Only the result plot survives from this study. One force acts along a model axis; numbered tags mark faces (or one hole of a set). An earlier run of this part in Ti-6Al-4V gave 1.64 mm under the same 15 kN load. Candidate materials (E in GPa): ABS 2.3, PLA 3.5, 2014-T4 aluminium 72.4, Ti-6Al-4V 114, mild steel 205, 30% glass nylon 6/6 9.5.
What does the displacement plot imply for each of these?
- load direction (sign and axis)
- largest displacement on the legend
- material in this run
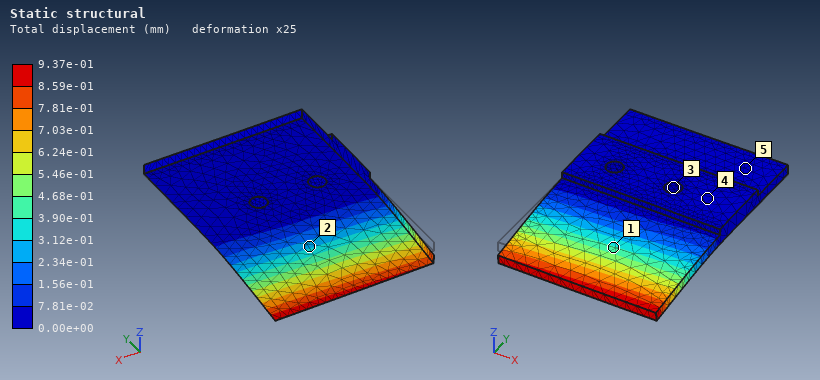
-Z
9.37e-01 mm
mild steel
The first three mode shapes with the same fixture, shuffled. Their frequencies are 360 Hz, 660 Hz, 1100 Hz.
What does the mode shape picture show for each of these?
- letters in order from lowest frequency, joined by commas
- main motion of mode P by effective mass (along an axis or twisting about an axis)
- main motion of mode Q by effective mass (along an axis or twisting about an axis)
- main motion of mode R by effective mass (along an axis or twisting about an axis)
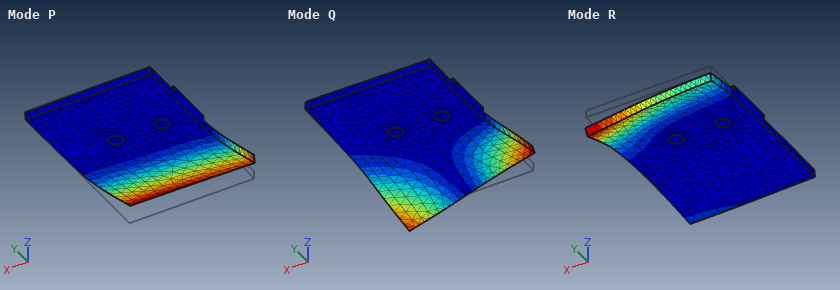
P, Q, R
along Z
twisting about Y
along Z
